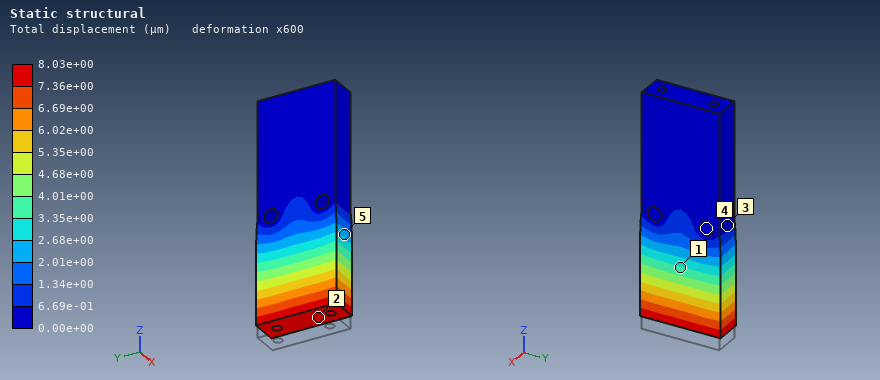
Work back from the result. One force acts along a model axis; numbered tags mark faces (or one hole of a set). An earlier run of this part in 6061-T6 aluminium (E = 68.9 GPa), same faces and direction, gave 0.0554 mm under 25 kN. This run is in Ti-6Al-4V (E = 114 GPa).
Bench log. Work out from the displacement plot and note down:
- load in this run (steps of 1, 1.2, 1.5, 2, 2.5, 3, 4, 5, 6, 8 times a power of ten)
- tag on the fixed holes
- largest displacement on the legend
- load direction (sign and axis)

6 kN
4
8.03e+00 µm
+Z
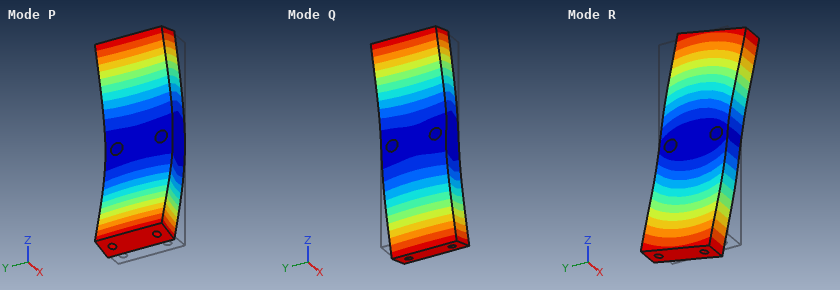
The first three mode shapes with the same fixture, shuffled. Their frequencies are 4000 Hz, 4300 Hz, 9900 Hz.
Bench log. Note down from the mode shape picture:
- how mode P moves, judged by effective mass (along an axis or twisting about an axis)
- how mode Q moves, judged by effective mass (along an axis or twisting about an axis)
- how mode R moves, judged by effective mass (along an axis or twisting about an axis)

along X
twisting about Y
twisting about X
